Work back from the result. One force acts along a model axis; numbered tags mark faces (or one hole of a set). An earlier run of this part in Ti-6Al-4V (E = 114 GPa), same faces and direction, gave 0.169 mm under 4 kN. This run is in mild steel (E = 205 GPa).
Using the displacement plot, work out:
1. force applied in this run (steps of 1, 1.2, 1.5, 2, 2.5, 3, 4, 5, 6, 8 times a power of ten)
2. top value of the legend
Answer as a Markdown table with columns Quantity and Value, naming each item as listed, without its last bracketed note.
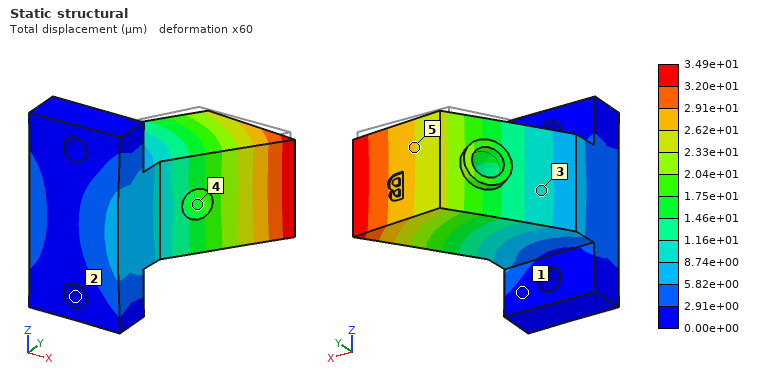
| Quantity | Value |
|---|---|
| force applied in this run | 1.5 kN |
| top value of the legend | 3.49e+01 µm |
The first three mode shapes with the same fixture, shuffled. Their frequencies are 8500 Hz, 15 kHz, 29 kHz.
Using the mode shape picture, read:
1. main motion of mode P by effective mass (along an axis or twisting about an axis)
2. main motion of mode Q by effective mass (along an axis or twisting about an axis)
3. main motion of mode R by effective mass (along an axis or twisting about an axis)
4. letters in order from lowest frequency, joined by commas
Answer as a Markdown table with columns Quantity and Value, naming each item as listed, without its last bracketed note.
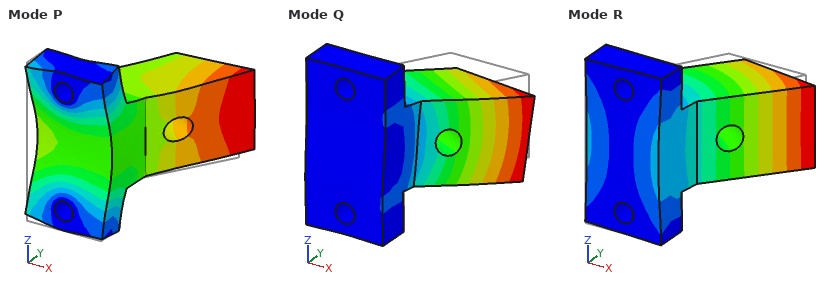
| Quantity | Value |
|---|---|
| main motion of mode P by effective mass | along Y |
| main motion of mode Q by effective mass | along Z |
| main motion of mode R by effective mass | along X |
| letters in order from lowest frequency, joined by commas | R, Q, P |
